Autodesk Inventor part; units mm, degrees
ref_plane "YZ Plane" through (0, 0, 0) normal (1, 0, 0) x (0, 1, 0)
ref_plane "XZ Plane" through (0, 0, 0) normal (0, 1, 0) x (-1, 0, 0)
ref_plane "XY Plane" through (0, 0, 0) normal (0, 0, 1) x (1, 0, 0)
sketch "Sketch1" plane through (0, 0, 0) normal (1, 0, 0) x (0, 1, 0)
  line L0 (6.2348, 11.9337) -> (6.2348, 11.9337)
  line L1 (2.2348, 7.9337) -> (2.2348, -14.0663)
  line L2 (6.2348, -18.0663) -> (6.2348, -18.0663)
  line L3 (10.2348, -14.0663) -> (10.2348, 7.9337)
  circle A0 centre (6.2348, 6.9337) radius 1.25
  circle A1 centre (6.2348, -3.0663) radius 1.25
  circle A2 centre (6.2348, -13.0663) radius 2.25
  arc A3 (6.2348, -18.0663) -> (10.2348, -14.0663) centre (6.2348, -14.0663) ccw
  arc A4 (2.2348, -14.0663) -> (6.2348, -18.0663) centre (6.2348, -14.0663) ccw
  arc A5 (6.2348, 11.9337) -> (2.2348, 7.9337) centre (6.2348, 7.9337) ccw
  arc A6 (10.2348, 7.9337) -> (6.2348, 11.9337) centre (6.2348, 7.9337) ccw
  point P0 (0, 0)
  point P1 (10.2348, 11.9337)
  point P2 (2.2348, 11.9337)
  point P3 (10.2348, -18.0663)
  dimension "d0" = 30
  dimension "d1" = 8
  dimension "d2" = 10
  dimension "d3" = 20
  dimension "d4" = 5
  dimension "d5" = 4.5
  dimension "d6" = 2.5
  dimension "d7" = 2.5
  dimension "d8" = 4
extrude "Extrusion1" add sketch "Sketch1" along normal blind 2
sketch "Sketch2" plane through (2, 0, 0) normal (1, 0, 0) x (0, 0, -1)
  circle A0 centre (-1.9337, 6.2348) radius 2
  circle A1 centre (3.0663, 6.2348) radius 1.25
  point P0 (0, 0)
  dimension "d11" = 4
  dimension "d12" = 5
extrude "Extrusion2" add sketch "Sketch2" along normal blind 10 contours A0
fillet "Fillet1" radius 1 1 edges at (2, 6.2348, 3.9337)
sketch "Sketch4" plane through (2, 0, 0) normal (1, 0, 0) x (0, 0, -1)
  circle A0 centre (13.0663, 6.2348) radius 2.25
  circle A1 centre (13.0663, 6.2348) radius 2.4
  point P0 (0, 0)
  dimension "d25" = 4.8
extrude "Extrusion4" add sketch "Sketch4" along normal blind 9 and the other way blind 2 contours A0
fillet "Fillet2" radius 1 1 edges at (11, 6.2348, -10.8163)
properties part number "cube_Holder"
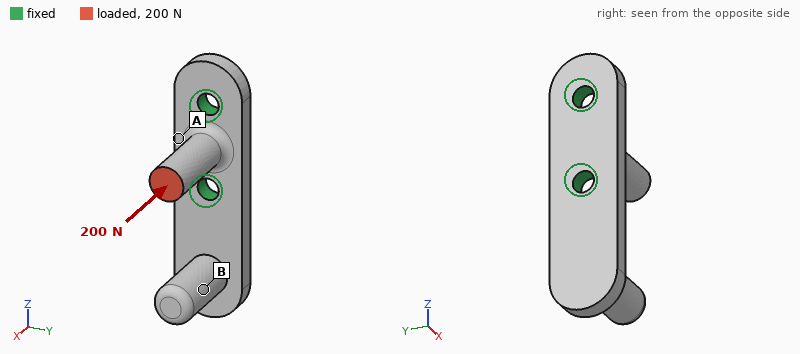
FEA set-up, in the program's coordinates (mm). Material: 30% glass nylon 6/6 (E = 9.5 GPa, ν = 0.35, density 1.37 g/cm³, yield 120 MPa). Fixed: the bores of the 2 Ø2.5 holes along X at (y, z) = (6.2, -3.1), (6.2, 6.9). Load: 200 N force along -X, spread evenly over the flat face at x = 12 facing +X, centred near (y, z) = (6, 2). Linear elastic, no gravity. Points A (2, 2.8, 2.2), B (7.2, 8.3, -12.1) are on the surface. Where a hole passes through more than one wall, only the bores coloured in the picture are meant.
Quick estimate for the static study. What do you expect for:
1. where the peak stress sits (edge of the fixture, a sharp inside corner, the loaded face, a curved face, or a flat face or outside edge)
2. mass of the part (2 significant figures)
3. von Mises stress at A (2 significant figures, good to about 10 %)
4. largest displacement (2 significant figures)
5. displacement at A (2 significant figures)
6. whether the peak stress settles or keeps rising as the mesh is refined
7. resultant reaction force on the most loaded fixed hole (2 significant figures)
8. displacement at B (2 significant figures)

edge of the fixture
0.96 g
13 MPa
30 µm
14 µm
keeps rising
100 N
7.0 µm
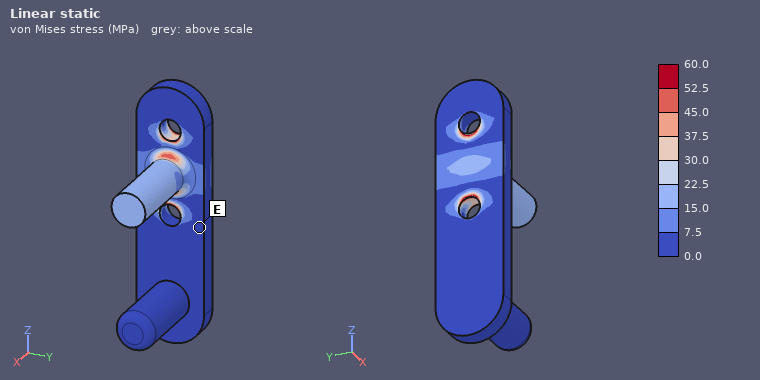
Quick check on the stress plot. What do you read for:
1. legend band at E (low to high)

0.0 to 7.5 MPa
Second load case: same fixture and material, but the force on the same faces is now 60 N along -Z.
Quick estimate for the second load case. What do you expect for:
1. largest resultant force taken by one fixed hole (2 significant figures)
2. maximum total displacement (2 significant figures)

99 N
0.22 mm
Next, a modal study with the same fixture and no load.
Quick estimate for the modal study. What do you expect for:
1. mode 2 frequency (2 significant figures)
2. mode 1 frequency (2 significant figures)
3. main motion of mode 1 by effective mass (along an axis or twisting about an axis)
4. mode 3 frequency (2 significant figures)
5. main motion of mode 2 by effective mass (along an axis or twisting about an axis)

4700 Hz
2800 Hz
along X
9500 Hz
along Y
